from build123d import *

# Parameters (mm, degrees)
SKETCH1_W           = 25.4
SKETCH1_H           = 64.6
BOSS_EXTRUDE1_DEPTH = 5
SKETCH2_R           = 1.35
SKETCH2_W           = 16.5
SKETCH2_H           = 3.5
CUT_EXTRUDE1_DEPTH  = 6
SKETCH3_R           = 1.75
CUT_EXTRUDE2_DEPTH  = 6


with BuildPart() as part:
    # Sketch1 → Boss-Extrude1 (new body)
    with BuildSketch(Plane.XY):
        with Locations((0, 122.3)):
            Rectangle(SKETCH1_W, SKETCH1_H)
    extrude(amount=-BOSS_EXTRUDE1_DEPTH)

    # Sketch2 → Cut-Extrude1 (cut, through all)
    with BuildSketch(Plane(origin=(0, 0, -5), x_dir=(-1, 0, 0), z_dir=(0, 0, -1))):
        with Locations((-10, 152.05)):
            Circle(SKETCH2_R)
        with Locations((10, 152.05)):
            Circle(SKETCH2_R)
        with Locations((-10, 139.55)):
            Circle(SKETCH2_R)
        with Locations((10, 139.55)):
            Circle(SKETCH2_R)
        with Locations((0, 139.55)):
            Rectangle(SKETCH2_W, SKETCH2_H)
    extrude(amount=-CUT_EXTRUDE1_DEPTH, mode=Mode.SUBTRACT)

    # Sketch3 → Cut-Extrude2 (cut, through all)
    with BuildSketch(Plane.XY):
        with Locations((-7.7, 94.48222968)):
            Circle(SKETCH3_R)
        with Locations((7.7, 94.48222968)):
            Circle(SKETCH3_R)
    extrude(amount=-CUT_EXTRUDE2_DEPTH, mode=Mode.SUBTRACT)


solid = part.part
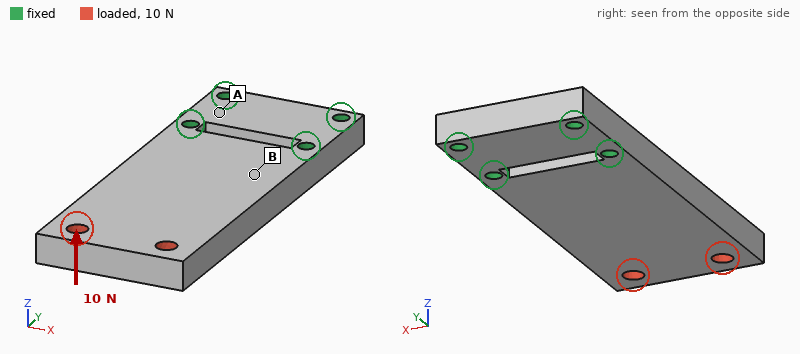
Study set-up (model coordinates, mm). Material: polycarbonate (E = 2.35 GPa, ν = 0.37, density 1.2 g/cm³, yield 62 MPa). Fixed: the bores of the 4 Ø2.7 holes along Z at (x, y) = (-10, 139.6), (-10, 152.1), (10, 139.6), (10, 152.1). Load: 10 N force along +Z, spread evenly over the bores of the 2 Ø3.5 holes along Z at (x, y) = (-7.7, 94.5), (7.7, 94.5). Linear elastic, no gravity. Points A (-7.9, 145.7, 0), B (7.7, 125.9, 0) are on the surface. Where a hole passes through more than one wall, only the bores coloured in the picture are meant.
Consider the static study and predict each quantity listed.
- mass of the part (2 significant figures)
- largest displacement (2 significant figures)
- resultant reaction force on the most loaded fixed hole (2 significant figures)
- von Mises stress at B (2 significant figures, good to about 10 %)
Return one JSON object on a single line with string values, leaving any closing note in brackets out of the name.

{"mass of the part": "9.2 g", "largest displacement": "0.79 mm", "resultant reaction force on the most loaded fixed hole": "5.5 N", "von Mises stress at B": "3.0 MPa"}
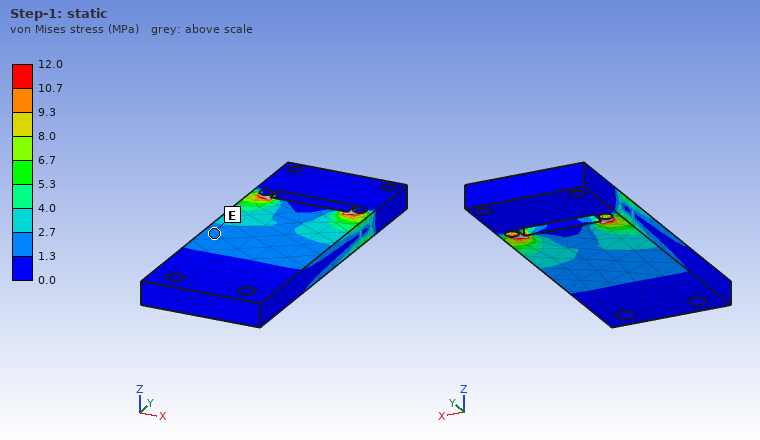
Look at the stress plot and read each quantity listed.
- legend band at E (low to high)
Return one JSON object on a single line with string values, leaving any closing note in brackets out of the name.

{"legend band at E": "1.3 to 2.7 MPa"}
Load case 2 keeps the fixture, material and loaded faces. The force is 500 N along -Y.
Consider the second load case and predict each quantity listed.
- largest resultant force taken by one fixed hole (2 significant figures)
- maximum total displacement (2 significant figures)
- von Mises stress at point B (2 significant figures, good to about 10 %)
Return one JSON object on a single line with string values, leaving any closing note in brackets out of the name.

{"largest resultant force taken by one fixed hole": "260 N", "maximum total displacement": "0.11 mm", "von Mises stress at point B": "4.3 MPa"}
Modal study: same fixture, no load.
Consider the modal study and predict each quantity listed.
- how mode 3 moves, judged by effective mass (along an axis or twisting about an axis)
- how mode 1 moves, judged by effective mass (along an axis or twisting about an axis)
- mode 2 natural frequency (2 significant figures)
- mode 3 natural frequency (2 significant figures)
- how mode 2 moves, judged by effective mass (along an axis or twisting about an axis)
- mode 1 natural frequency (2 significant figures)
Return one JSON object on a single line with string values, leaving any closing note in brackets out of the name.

{"how mode 3 moves, judged by effective mass": "along X", "how mode 1 moves, judged by effective mass": "along Z", "mode 2 natural frequency": "1800 Hz", "mode 3 natural frequency": "2000 Hz", "how mode 2 moves, judged by effective mass": "twisting about Y", "mode 1 natural frequency": "390 Hz"}
